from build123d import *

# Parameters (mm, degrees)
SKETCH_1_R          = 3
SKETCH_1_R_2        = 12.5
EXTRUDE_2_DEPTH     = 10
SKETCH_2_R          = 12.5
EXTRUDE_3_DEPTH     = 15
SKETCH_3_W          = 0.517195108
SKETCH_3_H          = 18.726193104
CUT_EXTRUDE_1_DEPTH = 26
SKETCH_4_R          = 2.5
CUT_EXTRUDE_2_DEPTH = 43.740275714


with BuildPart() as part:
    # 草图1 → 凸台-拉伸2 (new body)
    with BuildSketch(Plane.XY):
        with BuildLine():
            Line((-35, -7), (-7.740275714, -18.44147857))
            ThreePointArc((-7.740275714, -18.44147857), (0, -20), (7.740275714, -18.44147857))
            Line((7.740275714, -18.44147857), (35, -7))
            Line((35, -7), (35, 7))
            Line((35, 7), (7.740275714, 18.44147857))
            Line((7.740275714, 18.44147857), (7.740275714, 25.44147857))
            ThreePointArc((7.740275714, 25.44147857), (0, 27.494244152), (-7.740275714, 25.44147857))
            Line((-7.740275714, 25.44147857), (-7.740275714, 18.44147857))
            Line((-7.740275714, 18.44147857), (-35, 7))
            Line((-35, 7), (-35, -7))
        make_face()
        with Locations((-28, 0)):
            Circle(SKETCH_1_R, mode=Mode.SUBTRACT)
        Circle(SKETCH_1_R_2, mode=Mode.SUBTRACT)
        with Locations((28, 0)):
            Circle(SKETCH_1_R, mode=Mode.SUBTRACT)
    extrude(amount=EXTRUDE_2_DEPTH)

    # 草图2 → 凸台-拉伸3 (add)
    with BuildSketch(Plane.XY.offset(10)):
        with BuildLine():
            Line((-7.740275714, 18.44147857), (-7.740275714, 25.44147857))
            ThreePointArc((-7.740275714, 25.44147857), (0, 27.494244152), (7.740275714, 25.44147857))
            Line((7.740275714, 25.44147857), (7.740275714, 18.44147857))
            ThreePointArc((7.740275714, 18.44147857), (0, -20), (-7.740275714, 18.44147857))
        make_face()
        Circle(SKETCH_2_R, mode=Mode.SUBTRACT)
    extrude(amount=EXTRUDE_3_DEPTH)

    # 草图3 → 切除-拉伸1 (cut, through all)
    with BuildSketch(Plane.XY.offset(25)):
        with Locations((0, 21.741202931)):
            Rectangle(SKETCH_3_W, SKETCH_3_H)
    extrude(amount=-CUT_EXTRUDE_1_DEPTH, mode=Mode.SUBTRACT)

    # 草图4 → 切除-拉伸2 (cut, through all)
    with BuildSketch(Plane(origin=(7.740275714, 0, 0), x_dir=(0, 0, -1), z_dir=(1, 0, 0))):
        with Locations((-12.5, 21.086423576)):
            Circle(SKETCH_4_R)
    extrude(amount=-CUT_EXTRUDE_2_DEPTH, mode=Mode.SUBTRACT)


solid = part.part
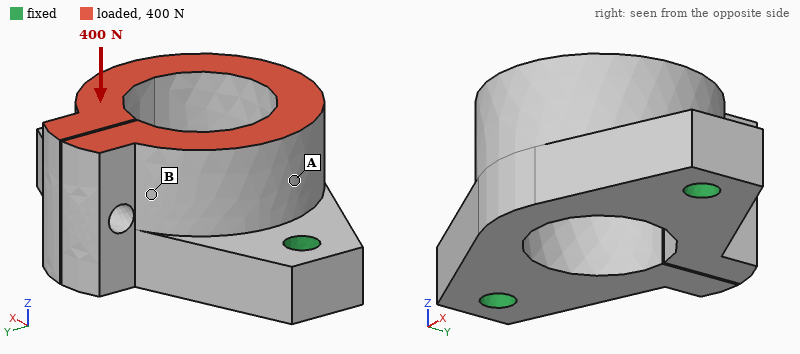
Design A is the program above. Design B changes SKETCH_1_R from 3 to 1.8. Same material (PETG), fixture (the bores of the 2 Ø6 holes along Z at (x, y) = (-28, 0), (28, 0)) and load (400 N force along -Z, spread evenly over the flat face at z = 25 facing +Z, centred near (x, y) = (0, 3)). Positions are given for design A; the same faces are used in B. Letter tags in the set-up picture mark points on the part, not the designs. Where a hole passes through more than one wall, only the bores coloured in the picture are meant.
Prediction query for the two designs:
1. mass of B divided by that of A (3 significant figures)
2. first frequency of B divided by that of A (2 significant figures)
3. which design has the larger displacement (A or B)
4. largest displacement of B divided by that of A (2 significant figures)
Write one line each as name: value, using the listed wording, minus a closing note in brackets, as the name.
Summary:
mass of B divided by that of A: 1.01
first frequency of B divided by that of A: 0.89
which design has the larger displacement: B
largest displacement of B divided by that of A: 1.2
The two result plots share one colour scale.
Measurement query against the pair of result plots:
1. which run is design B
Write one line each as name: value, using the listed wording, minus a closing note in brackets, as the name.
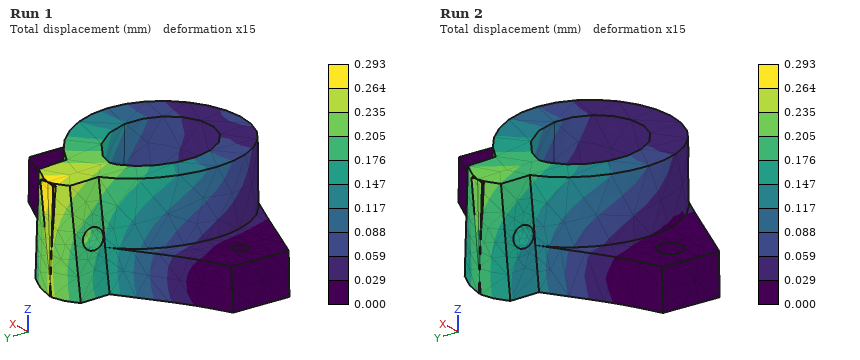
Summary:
which run is design B: Run 1
